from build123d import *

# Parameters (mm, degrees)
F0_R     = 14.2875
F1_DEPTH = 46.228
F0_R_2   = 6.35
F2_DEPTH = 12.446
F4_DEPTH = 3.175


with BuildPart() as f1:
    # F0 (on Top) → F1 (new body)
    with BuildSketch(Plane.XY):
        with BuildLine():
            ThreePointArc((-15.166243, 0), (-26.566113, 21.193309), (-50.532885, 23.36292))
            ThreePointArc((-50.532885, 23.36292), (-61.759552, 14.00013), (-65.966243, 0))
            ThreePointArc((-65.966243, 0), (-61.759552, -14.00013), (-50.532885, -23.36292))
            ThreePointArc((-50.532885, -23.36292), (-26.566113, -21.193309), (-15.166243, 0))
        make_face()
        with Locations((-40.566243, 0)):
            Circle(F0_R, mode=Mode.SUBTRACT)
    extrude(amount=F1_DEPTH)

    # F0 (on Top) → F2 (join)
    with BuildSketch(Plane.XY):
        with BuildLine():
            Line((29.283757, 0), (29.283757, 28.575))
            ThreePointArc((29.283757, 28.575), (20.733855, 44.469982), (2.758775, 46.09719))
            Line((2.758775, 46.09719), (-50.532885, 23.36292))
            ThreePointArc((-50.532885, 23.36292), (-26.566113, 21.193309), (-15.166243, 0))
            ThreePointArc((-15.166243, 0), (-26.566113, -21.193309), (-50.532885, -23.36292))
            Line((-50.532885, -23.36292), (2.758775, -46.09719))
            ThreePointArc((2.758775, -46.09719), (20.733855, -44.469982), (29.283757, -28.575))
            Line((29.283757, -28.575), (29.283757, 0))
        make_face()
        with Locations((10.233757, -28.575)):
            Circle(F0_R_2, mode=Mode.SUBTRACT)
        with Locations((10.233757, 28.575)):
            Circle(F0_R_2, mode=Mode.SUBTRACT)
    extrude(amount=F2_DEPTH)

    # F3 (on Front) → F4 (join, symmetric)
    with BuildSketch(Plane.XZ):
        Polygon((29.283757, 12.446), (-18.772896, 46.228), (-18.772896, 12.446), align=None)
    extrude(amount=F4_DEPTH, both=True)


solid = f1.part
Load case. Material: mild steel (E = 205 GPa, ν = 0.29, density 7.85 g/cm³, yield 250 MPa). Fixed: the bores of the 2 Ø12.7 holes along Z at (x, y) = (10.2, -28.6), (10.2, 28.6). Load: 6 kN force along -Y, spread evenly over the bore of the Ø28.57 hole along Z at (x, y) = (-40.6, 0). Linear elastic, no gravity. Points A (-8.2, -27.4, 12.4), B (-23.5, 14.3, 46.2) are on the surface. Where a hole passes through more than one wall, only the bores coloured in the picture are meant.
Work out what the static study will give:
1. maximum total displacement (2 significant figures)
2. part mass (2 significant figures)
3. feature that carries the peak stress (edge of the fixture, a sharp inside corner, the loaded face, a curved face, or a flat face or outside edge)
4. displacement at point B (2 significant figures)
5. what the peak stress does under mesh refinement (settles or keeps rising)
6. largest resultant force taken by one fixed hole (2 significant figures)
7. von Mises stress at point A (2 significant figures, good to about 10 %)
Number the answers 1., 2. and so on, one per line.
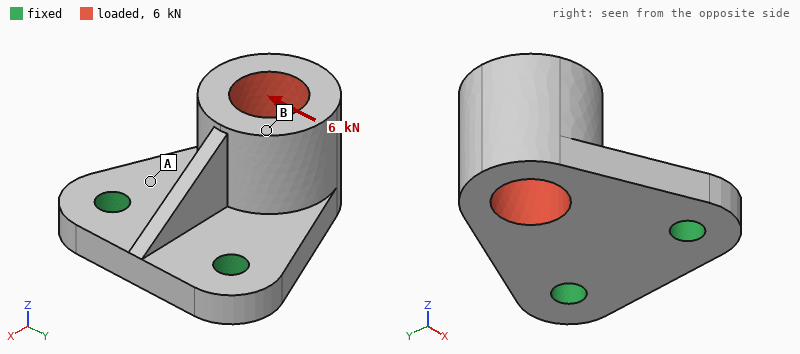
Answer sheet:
1. 25 µm
2. 960 g
3. edge of the fixture
4. 20 µm
5. keeps rising
6. 5.8 kN
7. 17 MPa
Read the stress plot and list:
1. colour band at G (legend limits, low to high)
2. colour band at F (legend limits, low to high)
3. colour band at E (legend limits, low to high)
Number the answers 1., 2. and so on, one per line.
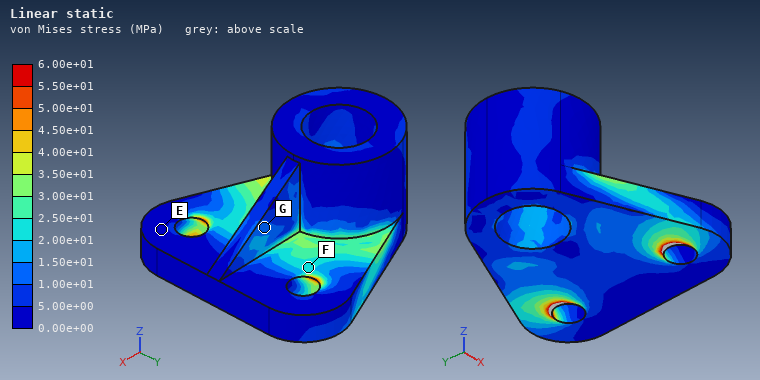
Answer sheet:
1. 1.00e+01 to 1.50e+01 MPa
2. 2.00e+01 to 2.50e+01 MPa
3. 0.00e+00 to 5.00e+00 MPa
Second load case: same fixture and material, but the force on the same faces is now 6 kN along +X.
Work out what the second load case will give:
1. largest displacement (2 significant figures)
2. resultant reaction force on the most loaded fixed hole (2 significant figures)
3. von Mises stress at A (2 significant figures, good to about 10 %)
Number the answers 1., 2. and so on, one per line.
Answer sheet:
1. 51 µm
2. 3.1 kN
3. 31 MPa
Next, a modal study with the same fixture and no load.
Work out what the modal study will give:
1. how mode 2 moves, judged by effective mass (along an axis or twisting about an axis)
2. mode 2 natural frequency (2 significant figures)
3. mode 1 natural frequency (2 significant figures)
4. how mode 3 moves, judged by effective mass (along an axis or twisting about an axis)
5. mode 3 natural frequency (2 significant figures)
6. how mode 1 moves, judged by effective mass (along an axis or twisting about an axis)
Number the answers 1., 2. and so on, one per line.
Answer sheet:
1. along Y
2. 3800 Hz
3. 1800 Hz
4. along Y
5. 7100 Hz
6. along Z
